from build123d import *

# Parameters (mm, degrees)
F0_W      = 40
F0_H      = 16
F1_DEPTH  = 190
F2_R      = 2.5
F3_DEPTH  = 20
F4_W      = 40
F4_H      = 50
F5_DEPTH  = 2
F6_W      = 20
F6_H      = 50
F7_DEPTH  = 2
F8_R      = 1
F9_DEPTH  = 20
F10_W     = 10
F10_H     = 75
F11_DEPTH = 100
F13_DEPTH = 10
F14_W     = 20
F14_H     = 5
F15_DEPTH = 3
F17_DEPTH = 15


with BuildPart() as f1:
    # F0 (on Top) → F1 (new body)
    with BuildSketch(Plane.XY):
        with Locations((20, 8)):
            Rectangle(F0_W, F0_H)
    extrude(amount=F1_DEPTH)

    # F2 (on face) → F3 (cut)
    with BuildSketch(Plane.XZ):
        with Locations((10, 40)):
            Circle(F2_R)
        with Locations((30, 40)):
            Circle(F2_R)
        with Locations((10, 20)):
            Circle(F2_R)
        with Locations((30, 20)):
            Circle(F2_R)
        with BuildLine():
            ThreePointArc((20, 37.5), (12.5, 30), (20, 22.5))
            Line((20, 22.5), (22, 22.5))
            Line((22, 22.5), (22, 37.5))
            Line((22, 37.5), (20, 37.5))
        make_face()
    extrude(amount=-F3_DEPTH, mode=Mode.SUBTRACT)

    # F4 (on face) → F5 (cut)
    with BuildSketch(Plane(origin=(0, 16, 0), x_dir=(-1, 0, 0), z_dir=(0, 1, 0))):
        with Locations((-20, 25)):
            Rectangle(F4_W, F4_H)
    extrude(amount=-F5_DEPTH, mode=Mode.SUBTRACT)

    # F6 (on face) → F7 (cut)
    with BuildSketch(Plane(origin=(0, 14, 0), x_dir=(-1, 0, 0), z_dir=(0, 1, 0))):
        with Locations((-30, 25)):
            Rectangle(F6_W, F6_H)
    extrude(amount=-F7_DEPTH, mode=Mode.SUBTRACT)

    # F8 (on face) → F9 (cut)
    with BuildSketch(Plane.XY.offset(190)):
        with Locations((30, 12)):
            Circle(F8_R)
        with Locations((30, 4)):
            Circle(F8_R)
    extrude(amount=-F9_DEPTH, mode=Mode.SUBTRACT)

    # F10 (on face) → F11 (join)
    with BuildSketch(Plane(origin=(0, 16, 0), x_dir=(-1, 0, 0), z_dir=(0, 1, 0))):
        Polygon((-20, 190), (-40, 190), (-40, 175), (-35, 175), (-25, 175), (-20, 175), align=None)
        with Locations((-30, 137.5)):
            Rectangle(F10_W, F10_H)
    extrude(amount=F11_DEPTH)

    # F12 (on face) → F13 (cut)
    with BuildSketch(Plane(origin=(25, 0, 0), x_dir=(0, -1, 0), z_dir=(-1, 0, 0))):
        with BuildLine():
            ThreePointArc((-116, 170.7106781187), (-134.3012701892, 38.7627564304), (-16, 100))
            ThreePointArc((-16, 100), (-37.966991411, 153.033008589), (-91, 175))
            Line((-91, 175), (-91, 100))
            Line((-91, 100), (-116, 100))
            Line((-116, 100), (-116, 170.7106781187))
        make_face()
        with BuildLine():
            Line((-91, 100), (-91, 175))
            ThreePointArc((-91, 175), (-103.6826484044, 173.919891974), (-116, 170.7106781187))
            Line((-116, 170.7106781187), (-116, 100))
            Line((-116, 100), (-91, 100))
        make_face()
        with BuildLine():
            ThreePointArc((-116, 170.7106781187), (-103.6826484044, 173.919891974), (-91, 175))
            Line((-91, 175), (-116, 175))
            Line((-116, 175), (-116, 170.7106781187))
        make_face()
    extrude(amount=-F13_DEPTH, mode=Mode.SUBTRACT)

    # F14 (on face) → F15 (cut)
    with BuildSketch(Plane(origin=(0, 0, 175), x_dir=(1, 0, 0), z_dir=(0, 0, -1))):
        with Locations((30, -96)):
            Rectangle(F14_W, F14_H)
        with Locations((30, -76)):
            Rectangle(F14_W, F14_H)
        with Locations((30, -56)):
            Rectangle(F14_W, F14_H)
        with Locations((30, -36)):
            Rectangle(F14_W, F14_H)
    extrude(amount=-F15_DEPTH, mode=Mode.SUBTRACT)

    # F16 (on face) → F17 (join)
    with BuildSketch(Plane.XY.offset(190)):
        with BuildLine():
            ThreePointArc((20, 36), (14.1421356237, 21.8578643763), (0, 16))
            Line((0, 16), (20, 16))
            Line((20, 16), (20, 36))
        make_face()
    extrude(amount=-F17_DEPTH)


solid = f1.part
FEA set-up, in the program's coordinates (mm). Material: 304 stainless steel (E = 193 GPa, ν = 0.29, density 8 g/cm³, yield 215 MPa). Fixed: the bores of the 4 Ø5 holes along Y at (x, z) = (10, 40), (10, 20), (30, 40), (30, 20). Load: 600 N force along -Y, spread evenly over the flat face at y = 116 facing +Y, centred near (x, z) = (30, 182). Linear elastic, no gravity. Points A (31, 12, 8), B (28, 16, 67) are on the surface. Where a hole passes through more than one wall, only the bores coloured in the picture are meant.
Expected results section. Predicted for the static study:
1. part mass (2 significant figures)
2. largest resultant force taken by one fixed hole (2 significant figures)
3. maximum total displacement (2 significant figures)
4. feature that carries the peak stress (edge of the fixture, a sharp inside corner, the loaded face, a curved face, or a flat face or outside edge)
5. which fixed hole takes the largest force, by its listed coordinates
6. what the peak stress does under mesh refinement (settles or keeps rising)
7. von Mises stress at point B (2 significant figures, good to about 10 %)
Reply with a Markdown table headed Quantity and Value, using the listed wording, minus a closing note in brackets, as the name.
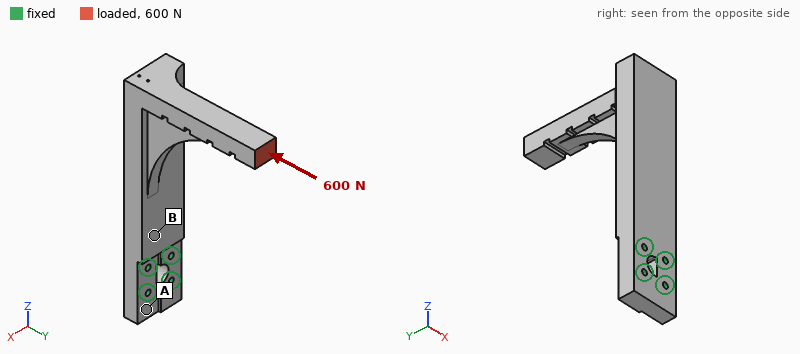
| Quantity | Value |
|---|---|
| part mass | 1.2 kg |
| largest resultant force taken by one fixed hole | 760 N |
| maximum total displacement | 0.40 mm |
| feature that carries the peak stress | edge of the fixture |
| which fixed hole takes the largest force, by its listed coordinates | (30, 40) |
| what the peak stress does under mesh refinement | keeps rising |
| von Mises stress at point B | 38 MPa |
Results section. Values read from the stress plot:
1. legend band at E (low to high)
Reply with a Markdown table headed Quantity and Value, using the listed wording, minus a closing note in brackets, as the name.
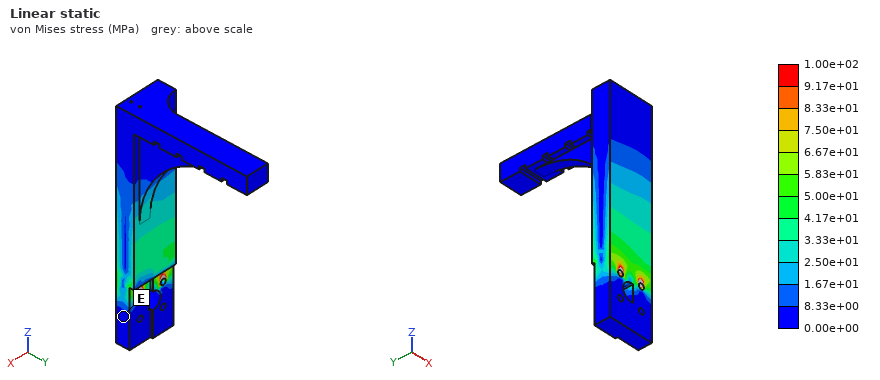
| Quantity | Value |
|---|---|
| legend band at E | 0.00e+00 to 8.33e+00 MPa |
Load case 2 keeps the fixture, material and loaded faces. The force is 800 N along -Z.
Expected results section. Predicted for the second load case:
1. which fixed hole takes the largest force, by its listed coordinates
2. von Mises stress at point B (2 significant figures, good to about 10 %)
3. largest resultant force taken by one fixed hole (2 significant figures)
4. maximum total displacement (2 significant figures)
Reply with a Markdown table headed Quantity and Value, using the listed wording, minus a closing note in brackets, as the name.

| Quantity | Value |
|---|---|
| which fixed hole takes the largest force, by its listed coordinates | (10, 40) |
| von Mises stress at point B | 50 MPa |
| largest resultant force taken by one fixed hole | 640 N |
| maximum total displacement | 0.62 mm |
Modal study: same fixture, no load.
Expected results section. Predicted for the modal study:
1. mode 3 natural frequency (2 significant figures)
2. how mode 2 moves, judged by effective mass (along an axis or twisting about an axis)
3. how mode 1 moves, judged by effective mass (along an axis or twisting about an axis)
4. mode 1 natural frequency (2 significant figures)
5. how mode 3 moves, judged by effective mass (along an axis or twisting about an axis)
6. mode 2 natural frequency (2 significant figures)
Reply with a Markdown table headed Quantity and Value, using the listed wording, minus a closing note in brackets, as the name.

| Quantity | Value |
|---|---|
| mode 3 natural frequency | 1200 Hz |
| how mode 2 moves, judged by effective mass | along X |
| how mode 1 moves, judged by effective mass | along Y |
| mode 1 natural frequency | 300 Hz |
| how mode 3 moves, judged by effective mass | along X |
| mode 2 natural frequency | 600 Hz |
